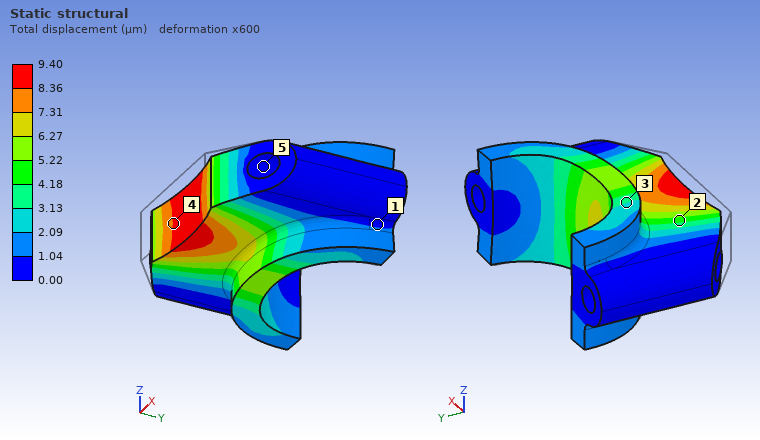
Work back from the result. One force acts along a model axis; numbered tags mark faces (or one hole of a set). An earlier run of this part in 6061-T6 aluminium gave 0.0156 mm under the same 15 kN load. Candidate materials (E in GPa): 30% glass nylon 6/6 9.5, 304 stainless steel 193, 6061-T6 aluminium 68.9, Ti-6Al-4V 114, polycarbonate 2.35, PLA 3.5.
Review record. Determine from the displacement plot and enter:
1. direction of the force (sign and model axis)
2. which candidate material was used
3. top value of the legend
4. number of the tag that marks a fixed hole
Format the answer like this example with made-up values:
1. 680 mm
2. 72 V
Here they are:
1. +Y
2. Ti-6Al-4V
3. 9.40 µm
4. 5
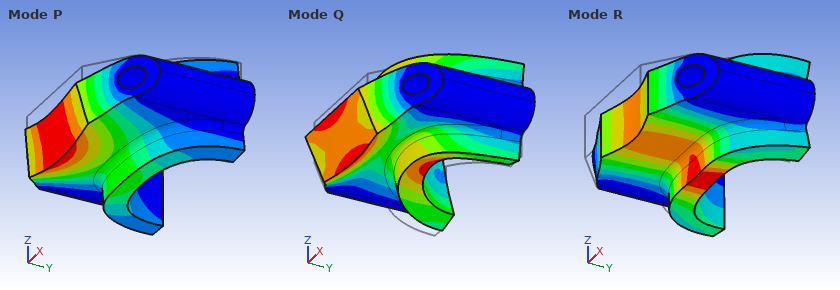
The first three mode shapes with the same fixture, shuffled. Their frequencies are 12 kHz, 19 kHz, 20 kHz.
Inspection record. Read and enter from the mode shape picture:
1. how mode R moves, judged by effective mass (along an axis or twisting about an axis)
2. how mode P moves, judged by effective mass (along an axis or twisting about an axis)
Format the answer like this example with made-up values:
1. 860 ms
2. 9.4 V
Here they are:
1. along Y
2. along Z
